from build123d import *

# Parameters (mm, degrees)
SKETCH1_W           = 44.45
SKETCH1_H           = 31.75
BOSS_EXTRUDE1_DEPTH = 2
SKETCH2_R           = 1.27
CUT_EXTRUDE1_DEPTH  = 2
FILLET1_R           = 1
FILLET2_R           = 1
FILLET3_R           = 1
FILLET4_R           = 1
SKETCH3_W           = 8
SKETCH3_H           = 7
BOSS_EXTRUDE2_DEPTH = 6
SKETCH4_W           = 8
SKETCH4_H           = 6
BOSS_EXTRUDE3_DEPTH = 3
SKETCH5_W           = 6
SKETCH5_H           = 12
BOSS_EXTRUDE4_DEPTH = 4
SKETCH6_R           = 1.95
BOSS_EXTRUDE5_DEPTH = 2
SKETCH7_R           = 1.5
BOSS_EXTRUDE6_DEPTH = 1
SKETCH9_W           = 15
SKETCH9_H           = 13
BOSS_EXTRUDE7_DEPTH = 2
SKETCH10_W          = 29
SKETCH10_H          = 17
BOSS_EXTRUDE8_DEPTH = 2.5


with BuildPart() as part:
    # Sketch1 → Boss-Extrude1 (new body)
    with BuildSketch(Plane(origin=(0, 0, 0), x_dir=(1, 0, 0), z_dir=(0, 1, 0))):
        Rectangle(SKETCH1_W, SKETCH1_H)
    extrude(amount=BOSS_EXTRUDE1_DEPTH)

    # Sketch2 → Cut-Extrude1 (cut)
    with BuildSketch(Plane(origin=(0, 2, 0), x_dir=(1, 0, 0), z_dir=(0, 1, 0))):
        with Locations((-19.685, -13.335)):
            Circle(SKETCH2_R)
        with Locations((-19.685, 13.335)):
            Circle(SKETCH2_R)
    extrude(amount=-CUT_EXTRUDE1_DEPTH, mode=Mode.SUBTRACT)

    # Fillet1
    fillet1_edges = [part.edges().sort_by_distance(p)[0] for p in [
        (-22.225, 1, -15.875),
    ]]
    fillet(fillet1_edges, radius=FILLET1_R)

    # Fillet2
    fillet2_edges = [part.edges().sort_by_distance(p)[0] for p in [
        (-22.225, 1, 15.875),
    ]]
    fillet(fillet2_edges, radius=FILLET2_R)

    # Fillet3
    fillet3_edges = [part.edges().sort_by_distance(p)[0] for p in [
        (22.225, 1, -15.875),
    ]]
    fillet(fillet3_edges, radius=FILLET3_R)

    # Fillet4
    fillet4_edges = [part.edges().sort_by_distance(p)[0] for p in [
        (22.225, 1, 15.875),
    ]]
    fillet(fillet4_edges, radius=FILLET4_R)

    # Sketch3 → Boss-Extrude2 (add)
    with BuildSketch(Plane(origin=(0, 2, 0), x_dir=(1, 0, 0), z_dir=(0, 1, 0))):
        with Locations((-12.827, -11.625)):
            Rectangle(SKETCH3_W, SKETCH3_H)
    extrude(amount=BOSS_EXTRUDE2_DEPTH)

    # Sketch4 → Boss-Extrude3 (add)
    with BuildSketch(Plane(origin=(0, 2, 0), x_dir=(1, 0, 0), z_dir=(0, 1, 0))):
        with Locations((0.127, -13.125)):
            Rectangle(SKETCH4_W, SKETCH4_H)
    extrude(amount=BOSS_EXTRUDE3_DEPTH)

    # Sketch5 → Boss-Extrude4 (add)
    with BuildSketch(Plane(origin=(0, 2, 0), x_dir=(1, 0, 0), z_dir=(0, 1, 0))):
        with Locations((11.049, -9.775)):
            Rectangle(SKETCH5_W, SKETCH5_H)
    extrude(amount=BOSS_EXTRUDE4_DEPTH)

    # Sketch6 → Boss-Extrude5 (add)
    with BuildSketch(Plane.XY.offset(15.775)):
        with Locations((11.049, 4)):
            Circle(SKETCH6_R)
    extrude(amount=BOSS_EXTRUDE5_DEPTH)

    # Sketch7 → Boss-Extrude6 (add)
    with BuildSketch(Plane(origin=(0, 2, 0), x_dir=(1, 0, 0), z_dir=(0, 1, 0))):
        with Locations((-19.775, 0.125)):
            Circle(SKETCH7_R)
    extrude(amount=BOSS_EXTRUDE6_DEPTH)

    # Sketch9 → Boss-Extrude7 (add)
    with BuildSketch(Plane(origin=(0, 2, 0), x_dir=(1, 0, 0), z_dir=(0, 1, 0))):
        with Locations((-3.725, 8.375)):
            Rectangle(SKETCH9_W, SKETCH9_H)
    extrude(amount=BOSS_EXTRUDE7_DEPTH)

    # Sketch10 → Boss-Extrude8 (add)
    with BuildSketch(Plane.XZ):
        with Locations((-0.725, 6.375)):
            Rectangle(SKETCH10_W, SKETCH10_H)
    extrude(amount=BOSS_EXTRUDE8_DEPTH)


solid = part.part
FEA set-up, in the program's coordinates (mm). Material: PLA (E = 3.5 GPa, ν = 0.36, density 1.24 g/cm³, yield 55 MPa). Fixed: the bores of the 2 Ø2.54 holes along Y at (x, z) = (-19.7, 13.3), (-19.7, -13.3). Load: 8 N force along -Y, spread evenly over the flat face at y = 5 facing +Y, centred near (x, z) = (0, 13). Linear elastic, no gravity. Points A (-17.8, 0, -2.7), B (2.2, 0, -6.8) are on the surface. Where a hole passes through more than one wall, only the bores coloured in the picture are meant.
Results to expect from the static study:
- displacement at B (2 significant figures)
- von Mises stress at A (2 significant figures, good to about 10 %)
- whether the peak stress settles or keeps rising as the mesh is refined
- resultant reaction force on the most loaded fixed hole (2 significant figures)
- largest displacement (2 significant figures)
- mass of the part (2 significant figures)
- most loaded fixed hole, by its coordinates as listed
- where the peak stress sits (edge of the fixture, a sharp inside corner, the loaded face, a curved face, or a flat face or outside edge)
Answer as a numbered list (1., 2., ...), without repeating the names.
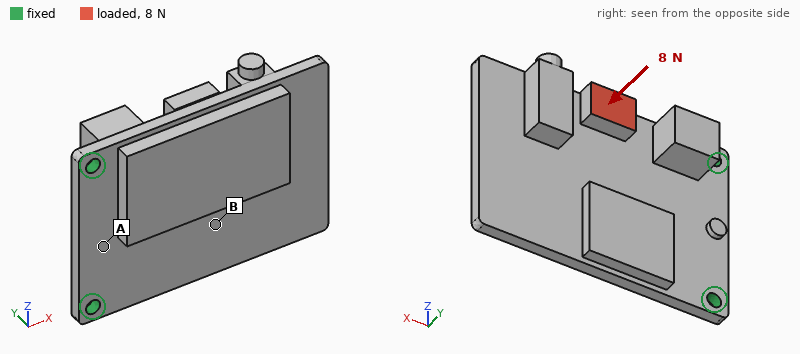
1. 0.26 mm
2. 2.6 MPa
3. keeps rising
4. 7.4 N
5. 0.59 mm
6. 6.5 g
7. (-19.7, 13.3)
8. edge of the fixture
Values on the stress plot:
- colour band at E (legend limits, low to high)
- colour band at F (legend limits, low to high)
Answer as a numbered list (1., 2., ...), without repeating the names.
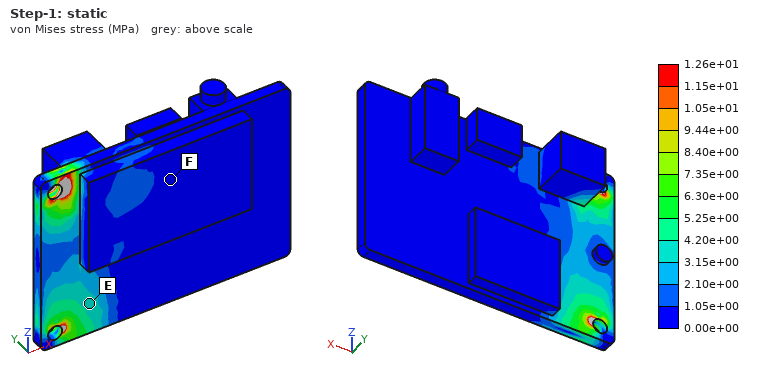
1. 3.15e+00 to 4.20e+00 MPa
2. 0.00e+00 to 1.05e+00 MPa
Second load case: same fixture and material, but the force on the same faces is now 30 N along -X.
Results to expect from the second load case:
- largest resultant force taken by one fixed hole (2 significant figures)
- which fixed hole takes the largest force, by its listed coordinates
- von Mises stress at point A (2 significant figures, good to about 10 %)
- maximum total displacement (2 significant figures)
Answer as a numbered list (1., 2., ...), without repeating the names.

1. 30 N
2. (-19.7, 13.3)
3. 2.1 MPa
4. 0.55 mm
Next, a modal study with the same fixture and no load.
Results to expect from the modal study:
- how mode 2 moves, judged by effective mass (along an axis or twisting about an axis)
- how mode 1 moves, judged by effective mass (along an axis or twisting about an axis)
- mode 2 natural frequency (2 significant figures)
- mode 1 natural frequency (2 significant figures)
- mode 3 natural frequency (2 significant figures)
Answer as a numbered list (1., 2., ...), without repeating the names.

1. twisting about X
2. along Y
3. 1600 Hz
4. 300 Hz
5. 2700 Hz
